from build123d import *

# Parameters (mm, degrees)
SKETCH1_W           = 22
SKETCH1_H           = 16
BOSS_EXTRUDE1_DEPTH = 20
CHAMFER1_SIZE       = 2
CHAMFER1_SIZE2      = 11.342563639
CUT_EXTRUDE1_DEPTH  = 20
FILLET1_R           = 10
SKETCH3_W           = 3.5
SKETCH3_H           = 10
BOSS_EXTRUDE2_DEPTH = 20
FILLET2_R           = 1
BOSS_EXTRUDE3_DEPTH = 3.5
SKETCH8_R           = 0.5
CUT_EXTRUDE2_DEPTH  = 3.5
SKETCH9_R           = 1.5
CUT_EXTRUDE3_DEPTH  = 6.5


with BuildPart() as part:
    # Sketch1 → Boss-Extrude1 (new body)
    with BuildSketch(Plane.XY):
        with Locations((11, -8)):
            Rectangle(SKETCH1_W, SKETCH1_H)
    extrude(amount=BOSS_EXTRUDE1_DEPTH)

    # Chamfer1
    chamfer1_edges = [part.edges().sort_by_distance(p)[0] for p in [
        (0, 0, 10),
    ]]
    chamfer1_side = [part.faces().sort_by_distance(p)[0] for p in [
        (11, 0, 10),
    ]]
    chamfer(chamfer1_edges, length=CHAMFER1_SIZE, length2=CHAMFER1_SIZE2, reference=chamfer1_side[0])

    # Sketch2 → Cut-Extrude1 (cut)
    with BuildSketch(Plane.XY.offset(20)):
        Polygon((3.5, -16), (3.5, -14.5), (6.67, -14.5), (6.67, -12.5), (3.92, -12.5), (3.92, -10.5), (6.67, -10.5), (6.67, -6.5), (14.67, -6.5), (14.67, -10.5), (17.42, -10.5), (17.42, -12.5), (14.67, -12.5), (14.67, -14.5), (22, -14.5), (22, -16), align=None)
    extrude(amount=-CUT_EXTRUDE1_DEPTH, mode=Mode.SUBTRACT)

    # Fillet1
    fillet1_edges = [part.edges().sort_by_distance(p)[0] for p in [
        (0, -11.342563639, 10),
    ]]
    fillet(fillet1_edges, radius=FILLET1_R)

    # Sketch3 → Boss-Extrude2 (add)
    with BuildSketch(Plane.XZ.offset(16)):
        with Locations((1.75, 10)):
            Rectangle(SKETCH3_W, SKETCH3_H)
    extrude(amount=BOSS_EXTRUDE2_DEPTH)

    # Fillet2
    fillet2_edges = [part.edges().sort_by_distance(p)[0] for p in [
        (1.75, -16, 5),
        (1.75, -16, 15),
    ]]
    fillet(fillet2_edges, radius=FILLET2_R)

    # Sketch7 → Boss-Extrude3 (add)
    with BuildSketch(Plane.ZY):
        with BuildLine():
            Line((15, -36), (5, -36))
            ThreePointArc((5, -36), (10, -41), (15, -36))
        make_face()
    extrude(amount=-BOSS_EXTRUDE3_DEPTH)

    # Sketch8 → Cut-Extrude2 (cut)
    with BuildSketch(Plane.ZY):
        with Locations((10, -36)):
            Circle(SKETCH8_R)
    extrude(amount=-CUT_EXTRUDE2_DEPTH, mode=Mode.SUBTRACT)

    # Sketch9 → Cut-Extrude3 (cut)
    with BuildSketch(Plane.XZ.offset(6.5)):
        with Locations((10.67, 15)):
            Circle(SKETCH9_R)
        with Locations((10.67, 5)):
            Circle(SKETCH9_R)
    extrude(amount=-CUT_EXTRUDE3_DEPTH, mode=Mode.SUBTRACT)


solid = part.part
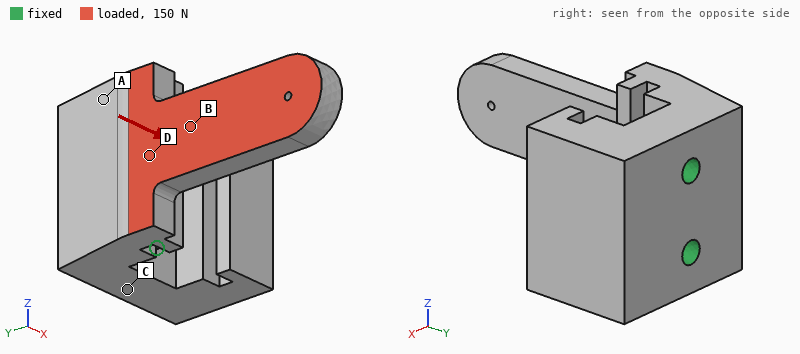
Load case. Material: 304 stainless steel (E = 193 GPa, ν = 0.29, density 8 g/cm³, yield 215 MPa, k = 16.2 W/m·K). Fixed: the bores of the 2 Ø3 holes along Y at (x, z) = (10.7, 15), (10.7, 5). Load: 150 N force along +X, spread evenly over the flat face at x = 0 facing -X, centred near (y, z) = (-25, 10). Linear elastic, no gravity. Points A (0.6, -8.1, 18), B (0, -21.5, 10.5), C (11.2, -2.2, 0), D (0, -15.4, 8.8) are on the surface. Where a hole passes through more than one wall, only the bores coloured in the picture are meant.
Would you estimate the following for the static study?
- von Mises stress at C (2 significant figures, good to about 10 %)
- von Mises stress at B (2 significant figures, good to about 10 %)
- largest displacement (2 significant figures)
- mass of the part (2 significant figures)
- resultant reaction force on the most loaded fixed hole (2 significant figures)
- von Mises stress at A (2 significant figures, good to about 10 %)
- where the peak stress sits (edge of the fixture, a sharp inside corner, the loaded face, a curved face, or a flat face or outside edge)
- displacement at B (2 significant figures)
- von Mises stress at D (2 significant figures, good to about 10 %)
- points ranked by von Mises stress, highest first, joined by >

6.8 MPa
39 MPa
73 µm
44 g
83 N
28 MPa
the loaded face
19 µm
56 MPa
D > B > A > C
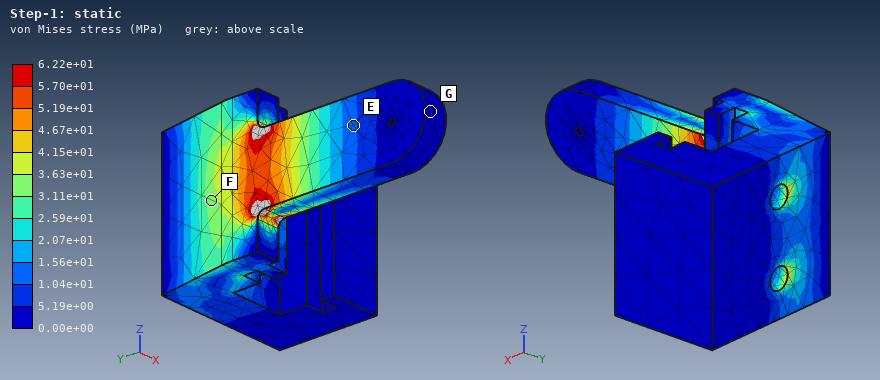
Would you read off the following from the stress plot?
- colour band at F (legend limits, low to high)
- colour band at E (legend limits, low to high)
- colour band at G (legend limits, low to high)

3.11e+01 to 3.63e+01 MPa
1.04e+01 to 1.56e+01 MPa
0.00e+00 to 5.19e+00 MPa
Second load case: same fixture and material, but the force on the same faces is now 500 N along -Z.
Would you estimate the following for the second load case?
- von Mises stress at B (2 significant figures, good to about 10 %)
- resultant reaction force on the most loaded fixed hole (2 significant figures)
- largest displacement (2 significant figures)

47 MPa
870 N
36 µm
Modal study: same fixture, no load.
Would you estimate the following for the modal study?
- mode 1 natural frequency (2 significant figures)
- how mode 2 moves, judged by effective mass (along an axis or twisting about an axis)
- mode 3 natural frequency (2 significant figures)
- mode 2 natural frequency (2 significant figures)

3100 Hz
along Z
13 kHz
7800 Hz
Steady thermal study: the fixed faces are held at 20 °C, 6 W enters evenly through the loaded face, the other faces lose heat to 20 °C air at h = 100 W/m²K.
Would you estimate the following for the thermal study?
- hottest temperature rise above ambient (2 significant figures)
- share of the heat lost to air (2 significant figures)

68 K
63 %
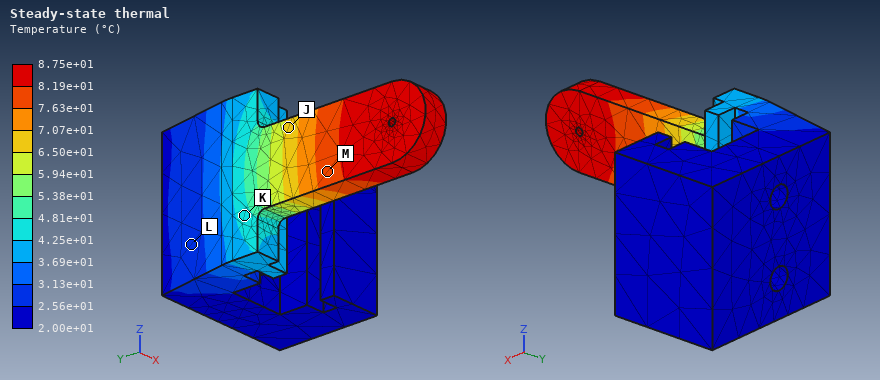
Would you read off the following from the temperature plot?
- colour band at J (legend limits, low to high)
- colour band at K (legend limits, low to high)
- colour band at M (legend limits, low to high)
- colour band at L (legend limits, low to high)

6.50e+01 to 7.07e+01 °C
4.25e+01 to 4.81e+01 °C
7.63e+01 to 8.19e+01 °C
2.56e+01 to 3.13e+01 °C
